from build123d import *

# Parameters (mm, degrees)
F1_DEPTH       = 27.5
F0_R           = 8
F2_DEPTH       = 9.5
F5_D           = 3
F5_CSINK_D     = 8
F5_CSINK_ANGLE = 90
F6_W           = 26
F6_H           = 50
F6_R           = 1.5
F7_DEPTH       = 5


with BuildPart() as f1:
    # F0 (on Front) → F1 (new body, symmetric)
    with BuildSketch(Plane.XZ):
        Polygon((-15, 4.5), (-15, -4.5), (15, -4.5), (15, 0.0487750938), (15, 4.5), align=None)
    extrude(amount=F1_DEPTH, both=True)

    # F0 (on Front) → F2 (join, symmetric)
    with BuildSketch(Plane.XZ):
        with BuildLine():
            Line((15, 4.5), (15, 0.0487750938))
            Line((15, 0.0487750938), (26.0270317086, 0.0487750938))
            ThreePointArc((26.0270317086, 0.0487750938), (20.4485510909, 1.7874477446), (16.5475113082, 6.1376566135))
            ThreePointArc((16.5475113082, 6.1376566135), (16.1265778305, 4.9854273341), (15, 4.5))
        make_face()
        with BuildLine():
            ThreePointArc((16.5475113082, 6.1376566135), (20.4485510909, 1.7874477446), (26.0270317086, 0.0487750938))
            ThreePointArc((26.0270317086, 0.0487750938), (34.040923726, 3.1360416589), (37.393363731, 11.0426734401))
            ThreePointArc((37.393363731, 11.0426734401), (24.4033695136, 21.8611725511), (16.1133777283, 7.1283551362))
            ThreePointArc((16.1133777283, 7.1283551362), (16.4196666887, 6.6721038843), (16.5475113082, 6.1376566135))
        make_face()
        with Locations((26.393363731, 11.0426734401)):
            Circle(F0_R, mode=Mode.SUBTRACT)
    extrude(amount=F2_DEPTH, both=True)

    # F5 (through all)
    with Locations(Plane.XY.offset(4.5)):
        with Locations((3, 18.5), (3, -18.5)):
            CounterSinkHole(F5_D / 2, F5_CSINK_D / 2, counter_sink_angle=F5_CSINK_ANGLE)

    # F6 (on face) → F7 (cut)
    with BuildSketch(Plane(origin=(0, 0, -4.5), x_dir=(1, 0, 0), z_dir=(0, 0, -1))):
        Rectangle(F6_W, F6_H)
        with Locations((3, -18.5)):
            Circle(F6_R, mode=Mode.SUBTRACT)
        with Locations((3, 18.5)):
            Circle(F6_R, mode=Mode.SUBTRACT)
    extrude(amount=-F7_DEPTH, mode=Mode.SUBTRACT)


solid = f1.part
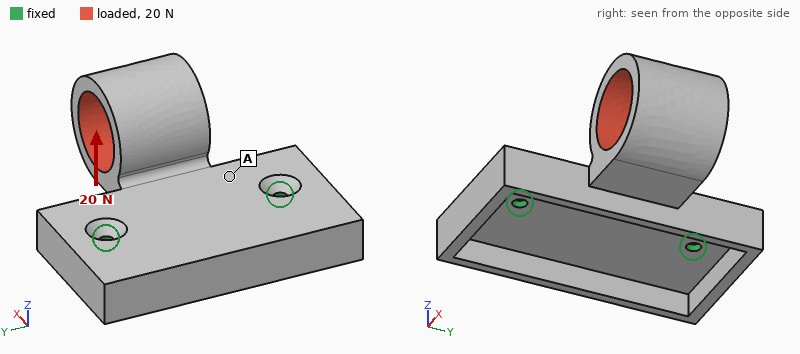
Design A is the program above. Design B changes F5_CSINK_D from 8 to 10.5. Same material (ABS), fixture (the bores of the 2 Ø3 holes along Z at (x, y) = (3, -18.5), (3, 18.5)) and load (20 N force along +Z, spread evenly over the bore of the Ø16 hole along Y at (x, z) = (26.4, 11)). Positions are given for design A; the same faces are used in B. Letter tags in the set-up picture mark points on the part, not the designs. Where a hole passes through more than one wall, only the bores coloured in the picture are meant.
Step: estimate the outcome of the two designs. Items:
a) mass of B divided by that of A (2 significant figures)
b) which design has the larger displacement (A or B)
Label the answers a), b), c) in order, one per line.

a) 0.99
b) B
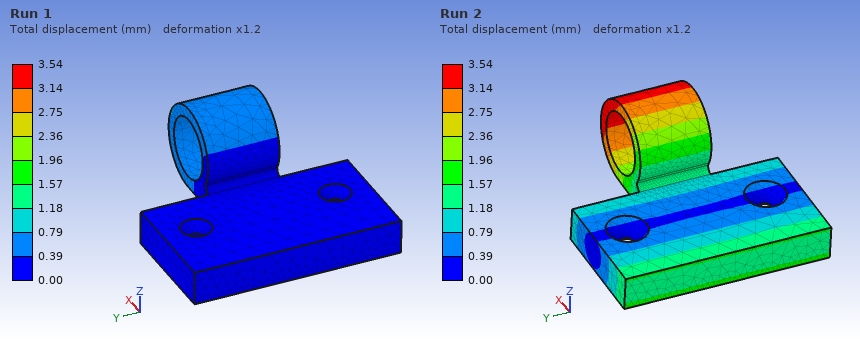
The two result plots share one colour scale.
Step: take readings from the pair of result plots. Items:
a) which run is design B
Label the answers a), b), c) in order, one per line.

a) Run 2
